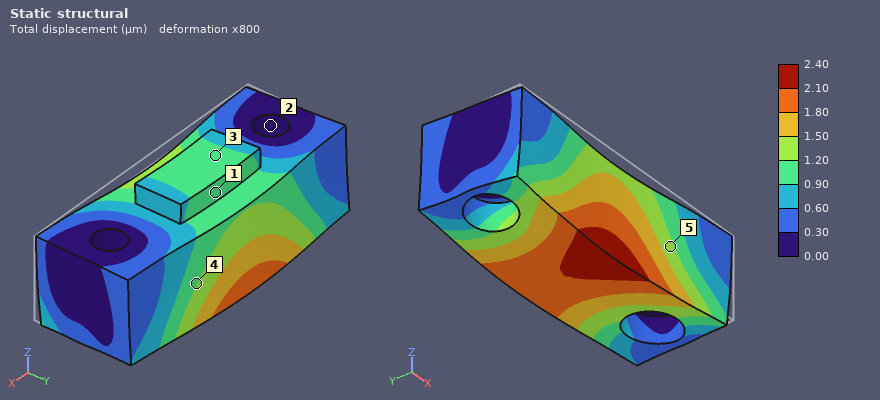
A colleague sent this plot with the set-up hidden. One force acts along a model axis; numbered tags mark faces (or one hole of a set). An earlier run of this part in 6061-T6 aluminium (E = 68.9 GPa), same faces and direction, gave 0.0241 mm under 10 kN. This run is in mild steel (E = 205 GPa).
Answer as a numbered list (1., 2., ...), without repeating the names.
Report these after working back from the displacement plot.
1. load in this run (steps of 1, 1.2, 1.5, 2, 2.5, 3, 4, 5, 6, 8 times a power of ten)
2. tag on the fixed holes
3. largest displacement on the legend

1. 3 kN
2. 2
3. 2.40 µm
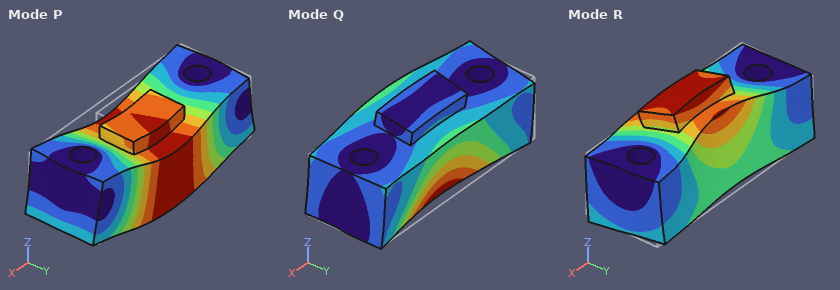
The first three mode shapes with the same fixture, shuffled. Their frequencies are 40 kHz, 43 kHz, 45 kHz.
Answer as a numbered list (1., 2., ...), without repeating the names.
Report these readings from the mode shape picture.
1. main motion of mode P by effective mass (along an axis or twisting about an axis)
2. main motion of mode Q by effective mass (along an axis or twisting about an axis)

1. along Z
2. along Y
